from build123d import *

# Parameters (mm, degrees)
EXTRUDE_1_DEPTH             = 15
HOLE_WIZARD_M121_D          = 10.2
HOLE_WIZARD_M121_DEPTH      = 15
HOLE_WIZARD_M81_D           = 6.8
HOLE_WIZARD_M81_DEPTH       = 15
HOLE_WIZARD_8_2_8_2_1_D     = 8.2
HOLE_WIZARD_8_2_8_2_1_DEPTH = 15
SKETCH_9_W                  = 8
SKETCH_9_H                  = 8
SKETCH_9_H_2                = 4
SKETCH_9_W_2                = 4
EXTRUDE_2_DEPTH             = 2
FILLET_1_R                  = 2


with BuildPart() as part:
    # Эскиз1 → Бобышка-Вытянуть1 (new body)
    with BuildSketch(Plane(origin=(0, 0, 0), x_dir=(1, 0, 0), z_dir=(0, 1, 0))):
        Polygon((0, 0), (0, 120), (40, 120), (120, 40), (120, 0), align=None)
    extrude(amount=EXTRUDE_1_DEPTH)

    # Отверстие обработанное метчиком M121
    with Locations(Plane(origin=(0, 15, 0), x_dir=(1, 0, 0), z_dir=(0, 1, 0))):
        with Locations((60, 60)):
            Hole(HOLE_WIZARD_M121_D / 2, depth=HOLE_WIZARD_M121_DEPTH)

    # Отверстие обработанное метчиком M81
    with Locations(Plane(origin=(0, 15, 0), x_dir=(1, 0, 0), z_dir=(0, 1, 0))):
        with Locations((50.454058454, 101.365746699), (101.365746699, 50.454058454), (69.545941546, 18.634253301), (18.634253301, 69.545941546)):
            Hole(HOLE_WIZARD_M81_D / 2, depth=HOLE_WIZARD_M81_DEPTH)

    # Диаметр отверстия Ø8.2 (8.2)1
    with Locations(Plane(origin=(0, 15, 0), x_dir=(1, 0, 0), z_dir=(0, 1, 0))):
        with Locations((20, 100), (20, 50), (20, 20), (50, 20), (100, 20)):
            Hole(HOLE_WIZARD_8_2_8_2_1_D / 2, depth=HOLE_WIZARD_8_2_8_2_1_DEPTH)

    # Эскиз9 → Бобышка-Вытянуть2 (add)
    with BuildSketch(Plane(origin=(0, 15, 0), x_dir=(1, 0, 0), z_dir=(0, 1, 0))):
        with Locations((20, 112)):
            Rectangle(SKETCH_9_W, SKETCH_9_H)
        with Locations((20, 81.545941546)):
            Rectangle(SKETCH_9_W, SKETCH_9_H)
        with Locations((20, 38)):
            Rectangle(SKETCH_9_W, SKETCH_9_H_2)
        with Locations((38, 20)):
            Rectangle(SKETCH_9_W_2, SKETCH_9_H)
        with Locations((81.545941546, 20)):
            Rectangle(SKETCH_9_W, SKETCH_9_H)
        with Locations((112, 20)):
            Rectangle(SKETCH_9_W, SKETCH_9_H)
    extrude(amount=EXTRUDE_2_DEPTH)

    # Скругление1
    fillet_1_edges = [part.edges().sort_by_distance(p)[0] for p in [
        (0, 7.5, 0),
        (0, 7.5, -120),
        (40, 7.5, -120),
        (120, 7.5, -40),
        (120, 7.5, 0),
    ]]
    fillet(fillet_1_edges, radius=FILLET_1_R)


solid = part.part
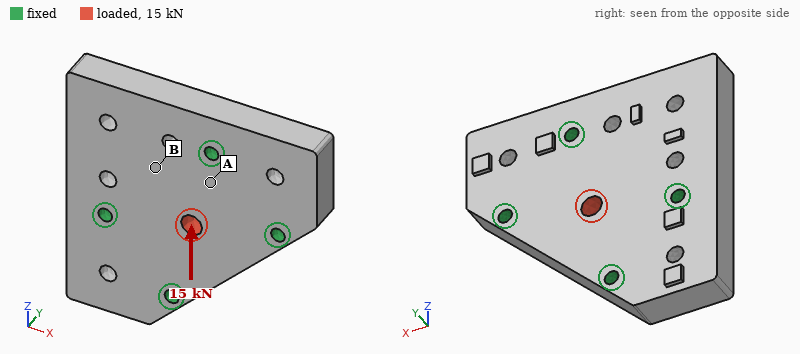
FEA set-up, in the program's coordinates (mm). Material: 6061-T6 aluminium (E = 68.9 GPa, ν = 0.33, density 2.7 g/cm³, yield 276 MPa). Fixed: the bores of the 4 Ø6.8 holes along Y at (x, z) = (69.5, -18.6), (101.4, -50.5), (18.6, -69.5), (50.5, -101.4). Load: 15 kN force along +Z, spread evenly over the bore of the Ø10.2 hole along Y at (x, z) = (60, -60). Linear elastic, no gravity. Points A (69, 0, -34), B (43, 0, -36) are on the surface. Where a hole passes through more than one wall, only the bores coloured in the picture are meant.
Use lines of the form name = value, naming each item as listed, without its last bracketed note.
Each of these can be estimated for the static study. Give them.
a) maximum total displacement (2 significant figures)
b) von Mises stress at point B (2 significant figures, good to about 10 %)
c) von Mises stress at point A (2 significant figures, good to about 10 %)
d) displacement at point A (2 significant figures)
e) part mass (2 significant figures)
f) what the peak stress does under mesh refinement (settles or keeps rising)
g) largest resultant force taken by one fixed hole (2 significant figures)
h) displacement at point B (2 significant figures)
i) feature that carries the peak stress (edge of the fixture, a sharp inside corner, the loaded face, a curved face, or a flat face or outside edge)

maximum total displacement = 12 µm
von Mises stress at point B = 6.8 MPa
von Mises stress at point A = 19 MPa
displacement at point A = 3.6 µm
part mass = 440 g
what the peak stress does under mesh refinement = keeps rising
largest resultant force taken by one fixed hole = 5.6 kN
displacement at point B = 5.4 µm
feature that carries the peak stress = a sharp inside corner
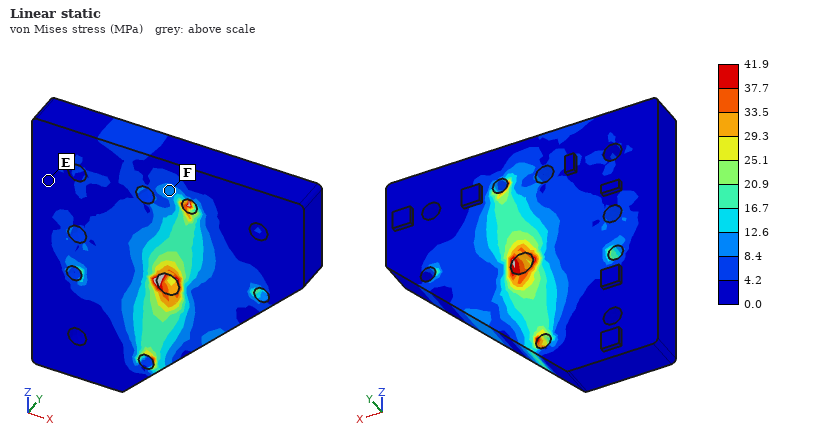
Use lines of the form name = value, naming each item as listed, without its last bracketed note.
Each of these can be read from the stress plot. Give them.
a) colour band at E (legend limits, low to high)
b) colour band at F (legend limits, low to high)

colour band at E = 0.0 to 4.2 MPa
colour band at F = 8.4 to 12.6 MPa
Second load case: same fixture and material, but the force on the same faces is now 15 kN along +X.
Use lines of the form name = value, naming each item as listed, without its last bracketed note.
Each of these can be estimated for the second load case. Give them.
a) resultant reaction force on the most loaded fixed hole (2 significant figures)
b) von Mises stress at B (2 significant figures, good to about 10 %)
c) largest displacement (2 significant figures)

resultant reaction force on the most loaded fixed hole = 5.6 kN
von Mises stress at B = 6.2 MPa
largest displacement = 12 µm
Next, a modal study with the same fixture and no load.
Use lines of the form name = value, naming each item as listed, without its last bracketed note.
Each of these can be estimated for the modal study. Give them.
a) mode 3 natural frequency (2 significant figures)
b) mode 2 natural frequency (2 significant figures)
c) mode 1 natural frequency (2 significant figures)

mode 3 natural frequency = 7200 Hz
mode 2 natural frequency = 7100 Hz
mode 1 natural frequency = 4200 Hz
